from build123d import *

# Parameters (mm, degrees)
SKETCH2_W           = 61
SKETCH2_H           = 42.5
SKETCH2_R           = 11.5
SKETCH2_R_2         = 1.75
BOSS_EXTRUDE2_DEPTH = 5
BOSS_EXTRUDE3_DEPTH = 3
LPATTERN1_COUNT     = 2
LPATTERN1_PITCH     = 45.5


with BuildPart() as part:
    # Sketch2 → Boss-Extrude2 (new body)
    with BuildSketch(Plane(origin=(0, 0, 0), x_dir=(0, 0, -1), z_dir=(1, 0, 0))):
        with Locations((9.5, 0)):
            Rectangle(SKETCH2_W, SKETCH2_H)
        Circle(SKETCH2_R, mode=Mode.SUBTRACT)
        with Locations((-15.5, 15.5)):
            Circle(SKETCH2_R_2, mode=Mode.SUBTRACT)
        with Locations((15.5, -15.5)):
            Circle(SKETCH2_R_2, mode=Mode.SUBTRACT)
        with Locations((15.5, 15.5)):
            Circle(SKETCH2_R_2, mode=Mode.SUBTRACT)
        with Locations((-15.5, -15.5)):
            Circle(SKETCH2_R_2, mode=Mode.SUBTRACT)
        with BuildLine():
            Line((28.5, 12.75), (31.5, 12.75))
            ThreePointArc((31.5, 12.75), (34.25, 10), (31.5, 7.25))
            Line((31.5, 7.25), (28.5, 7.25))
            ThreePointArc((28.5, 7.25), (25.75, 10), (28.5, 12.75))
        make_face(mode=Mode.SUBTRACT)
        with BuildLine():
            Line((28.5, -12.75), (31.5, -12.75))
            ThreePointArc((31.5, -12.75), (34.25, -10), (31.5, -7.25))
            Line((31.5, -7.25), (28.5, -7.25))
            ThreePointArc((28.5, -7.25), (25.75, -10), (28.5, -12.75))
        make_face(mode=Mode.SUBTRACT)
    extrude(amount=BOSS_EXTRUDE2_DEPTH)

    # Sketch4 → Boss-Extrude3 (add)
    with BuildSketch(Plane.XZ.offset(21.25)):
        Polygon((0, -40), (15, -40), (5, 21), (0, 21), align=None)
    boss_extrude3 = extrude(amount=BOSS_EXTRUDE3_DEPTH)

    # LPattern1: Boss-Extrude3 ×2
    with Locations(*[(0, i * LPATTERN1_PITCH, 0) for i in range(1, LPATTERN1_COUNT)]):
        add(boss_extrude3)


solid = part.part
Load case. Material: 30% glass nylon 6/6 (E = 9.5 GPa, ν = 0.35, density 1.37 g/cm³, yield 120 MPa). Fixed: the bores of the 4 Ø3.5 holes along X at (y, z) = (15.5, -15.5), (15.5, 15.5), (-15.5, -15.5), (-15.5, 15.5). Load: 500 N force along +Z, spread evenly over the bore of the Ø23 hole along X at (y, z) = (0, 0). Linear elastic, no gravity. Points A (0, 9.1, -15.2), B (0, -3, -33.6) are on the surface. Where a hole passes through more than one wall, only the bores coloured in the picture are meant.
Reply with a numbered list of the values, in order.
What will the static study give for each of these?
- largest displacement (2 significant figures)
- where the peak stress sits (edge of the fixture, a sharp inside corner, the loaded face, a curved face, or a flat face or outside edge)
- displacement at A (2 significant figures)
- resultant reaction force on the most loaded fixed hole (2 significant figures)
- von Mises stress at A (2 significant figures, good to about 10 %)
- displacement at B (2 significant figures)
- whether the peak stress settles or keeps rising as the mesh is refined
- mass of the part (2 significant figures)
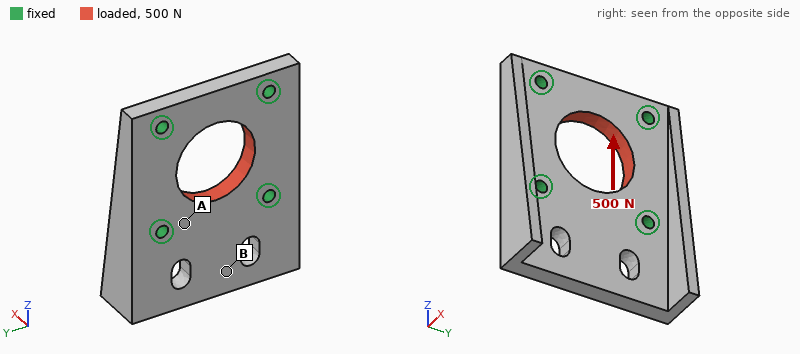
1. 7.0 µm
2. edge of the fixture
3. 1.9 µm
4. 130 N
5. 1.2 MPa
6. 2.0 µm
7. keeps rising
8. 19 g
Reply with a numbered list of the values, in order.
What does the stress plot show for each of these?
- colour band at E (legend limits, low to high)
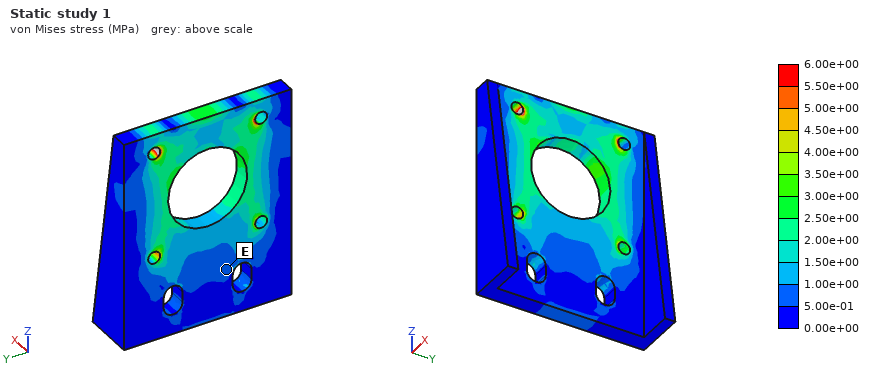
1. 5.00e-01 to 1.00e+00 MPa
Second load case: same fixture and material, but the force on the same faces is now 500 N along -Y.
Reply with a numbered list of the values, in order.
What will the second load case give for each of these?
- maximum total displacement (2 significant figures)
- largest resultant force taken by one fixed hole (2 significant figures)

1. 5.2 µm
2. 130 N
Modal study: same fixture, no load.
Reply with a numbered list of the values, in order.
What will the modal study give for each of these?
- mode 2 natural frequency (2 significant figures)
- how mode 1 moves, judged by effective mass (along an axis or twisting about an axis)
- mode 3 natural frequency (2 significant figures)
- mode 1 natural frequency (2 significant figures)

1. 4500 Hz
2. along X
3. 5900 Hz
4. 3600 Hz
